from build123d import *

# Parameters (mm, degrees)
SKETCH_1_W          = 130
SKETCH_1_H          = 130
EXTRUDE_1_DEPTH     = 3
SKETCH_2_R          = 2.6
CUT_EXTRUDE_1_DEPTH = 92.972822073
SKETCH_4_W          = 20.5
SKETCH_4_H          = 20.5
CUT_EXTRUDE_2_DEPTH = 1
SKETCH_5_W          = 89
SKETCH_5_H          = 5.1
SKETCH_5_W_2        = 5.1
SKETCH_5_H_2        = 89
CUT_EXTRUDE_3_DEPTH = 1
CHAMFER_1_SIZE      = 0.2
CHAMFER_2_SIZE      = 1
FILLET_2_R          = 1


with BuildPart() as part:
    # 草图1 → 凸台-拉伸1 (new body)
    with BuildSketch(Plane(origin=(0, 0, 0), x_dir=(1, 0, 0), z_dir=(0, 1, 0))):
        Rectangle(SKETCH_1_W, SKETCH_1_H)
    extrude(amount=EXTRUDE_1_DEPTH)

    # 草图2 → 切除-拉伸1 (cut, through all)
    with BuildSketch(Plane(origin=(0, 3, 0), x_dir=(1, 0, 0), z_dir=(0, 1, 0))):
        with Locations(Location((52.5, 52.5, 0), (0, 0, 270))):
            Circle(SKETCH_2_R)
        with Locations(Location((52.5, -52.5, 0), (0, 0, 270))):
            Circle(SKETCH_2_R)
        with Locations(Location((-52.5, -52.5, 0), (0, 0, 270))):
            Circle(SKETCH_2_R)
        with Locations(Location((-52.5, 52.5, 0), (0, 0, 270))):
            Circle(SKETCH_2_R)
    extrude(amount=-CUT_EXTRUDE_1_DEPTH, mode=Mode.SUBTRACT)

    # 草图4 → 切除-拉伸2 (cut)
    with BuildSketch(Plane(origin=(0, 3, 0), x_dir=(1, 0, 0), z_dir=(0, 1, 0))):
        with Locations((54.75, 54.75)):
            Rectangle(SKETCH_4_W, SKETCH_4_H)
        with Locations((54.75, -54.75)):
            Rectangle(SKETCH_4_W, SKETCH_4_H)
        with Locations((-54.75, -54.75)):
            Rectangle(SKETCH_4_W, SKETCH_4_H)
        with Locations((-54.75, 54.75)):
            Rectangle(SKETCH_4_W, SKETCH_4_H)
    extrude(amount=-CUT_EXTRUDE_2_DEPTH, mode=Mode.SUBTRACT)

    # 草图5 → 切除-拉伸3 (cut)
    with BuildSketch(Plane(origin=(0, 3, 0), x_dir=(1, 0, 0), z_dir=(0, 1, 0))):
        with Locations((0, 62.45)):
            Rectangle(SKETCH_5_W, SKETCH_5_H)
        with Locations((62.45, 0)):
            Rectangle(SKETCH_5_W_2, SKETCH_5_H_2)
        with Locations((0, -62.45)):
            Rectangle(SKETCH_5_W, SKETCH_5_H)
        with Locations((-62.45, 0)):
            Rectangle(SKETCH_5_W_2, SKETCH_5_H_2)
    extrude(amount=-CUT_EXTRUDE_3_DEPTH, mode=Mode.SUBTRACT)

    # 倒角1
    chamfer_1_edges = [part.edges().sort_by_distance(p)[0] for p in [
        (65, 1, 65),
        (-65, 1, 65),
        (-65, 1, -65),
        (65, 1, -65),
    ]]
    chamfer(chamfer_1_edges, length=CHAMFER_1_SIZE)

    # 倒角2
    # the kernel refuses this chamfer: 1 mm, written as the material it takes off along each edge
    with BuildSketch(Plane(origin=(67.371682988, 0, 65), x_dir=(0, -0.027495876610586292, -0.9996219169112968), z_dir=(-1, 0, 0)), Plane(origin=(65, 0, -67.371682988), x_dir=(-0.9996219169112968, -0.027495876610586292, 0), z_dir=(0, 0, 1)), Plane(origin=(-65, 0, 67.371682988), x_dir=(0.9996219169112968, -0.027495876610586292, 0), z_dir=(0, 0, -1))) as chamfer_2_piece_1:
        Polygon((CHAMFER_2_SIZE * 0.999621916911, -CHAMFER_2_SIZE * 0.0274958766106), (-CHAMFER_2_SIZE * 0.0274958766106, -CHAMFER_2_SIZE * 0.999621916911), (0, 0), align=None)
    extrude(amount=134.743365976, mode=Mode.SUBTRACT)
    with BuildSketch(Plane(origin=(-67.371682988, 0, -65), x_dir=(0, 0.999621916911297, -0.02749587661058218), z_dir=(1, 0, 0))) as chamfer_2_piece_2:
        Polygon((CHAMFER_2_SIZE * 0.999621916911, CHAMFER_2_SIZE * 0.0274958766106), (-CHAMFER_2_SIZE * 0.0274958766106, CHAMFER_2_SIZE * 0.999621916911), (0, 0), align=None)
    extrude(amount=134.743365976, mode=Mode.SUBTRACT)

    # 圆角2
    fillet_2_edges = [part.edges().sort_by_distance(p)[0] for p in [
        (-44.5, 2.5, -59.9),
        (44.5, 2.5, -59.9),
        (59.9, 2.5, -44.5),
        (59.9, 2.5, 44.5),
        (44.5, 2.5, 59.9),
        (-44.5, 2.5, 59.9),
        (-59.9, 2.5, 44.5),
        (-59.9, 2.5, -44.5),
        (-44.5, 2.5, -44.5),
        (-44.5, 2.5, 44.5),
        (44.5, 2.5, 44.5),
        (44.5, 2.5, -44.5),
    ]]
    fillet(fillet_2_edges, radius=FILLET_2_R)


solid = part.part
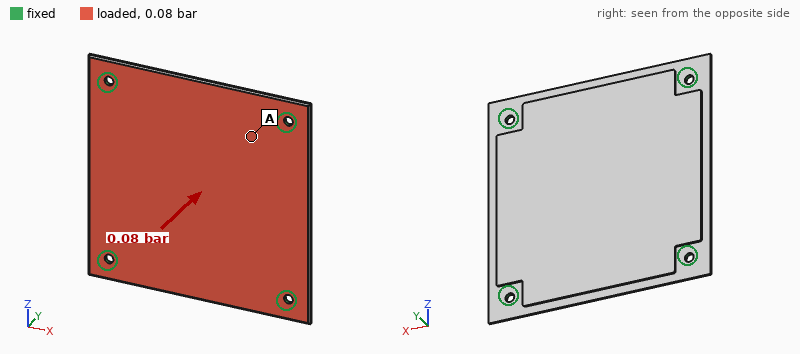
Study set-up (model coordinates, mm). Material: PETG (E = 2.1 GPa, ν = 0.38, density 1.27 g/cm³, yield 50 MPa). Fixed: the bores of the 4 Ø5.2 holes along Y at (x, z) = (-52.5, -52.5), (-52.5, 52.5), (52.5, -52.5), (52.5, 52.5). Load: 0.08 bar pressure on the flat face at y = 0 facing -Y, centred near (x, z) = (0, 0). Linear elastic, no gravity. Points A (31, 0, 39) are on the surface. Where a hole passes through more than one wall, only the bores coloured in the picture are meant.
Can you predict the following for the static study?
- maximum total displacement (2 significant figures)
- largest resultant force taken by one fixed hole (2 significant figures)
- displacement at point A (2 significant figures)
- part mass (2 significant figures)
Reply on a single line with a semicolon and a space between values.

1.8 mm; 78 N; 0.86 mm; 59 g
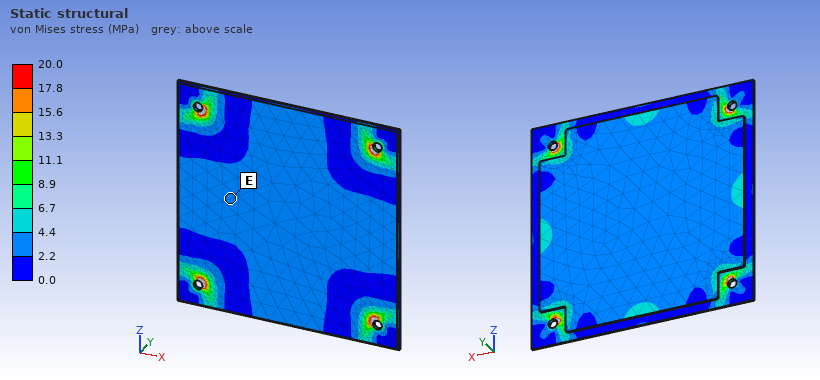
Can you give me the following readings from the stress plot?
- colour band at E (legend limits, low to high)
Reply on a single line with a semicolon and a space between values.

2.2 to 4.4 MPa
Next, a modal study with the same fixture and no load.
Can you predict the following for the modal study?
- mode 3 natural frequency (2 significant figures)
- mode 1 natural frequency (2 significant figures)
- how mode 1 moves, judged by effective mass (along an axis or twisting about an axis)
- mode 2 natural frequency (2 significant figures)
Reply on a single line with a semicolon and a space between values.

340 Hz; 210 Hz; along Y; 340 Hz
